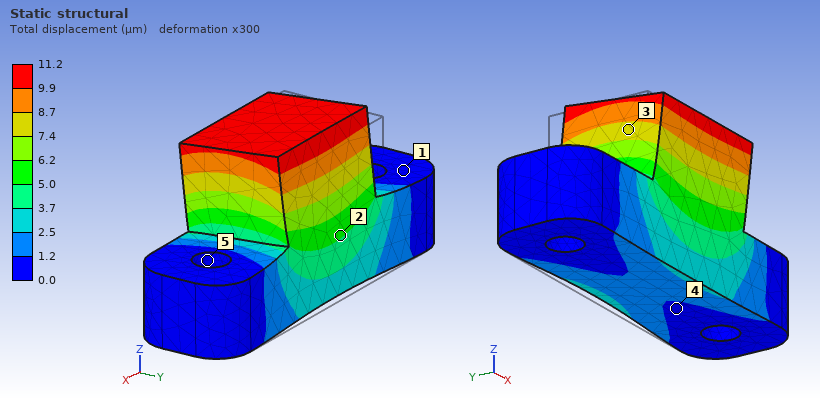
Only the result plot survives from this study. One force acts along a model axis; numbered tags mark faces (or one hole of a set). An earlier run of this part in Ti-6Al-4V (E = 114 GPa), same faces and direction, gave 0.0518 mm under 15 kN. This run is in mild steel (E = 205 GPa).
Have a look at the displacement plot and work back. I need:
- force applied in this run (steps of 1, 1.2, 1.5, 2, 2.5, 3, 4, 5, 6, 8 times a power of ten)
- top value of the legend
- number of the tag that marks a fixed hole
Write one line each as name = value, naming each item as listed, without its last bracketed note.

force applied in this run = 6 kN
top value of the legend = 11.2 µm
number of the tag that marks a fixed hole = 5
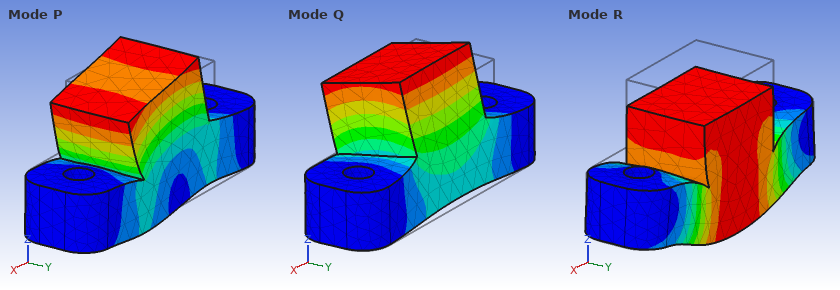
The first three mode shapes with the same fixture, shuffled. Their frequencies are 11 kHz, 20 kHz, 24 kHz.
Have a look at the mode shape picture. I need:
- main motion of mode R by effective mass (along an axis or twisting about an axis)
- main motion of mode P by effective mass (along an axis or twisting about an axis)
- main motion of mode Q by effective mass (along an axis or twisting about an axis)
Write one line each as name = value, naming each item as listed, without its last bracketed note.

main motion of mode R by effective mass = along Z
main motion of mode P by effective mass = along X
main motion of mode Q by effective mass = along Y
